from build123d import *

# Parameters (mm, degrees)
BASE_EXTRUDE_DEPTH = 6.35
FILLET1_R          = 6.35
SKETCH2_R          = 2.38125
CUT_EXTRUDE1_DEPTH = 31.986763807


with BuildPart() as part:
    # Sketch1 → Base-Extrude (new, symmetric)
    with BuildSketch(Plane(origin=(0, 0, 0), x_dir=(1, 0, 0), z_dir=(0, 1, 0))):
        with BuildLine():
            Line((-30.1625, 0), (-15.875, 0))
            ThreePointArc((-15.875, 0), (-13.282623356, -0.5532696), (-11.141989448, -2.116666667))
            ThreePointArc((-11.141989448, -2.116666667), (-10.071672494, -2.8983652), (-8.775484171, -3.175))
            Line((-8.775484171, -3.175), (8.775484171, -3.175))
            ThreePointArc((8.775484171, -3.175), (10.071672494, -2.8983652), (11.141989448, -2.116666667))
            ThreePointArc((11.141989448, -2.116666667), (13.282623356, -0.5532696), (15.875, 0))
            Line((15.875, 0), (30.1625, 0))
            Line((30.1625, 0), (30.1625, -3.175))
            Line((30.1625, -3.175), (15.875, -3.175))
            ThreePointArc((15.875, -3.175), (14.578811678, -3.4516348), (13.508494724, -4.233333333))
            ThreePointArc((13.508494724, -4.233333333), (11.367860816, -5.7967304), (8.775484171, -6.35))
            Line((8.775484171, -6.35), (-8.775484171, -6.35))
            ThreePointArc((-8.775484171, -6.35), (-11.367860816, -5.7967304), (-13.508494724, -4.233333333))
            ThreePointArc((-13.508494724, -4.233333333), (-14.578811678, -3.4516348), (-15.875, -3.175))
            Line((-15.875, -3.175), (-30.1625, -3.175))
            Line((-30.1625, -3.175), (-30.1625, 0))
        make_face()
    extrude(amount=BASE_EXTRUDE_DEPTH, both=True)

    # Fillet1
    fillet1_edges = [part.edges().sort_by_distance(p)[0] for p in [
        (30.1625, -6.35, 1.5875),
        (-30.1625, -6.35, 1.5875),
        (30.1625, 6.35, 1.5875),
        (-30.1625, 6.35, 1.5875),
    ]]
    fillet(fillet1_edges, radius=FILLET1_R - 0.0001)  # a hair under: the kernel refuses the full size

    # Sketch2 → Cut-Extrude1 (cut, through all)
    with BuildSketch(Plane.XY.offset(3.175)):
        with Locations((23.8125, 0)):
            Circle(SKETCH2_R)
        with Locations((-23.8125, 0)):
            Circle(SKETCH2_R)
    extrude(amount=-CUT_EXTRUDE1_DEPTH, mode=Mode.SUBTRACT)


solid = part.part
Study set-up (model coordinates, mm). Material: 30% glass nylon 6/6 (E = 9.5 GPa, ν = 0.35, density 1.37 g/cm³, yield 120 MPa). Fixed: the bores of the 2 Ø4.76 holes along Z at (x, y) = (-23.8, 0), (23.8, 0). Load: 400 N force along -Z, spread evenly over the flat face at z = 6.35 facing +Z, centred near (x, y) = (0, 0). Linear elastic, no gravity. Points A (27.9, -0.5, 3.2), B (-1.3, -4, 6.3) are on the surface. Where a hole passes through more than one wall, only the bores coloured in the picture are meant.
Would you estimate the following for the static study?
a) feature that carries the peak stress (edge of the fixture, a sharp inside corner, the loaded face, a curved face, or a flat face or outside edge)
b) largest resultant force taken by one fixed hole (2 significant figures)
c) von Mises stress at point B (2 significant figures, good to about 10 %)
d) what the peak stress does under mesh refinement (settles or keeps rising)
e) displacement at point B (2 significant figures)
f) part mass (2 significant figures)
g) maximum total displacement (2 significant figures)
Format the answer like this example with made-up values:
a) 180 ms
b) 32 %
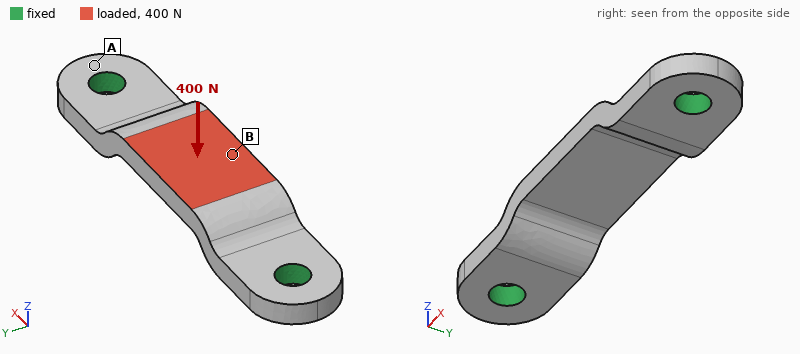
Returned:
a) edge of the fixture
b) 560 N
c) 45 MPa
d) keeps rising
e) 0.22 mm
f) 3.1 g
g) 0.23 mm
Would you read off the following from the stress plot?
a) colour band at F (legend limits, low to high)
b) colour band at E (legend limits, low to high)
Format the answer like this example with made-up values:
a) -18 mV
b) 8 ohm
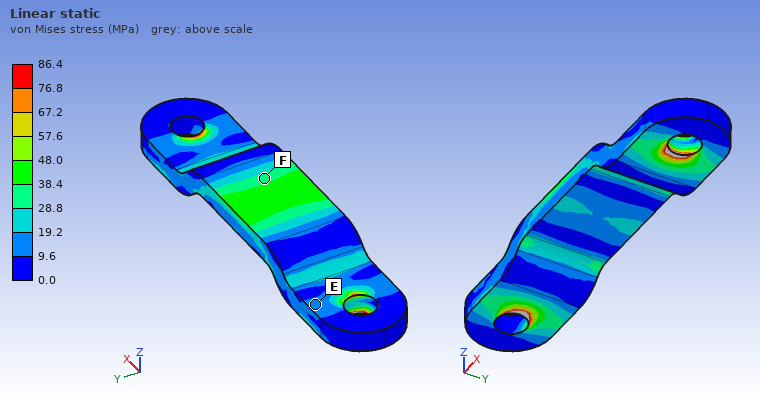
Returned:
a) 28.8 to 38.4 MPa
b) 9.6 to 19.2 MPa
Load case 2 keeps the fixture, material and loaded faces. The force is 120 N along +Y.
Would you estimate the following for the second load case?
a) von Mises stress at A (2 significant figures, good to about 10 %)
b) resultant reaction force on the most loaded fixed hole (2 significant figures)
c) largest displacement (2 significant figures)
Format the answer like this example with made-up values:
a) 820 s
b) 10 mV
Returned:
a) 2.7 MPa
b) 60 N
c) 72 µm
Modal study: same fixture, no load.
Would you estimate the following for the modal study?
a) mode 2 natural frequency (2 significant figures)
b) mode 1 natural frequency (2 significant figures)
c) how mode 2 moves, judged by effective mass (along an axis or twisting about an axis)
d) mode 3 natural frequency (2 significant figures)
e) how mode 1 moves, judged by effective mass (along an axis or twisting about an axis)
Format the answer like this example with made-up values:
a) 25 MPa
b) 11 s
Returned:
a) 6700 Hz
b) 6300 Hz
c) along Y
d) 10 kHz
e) along Z
